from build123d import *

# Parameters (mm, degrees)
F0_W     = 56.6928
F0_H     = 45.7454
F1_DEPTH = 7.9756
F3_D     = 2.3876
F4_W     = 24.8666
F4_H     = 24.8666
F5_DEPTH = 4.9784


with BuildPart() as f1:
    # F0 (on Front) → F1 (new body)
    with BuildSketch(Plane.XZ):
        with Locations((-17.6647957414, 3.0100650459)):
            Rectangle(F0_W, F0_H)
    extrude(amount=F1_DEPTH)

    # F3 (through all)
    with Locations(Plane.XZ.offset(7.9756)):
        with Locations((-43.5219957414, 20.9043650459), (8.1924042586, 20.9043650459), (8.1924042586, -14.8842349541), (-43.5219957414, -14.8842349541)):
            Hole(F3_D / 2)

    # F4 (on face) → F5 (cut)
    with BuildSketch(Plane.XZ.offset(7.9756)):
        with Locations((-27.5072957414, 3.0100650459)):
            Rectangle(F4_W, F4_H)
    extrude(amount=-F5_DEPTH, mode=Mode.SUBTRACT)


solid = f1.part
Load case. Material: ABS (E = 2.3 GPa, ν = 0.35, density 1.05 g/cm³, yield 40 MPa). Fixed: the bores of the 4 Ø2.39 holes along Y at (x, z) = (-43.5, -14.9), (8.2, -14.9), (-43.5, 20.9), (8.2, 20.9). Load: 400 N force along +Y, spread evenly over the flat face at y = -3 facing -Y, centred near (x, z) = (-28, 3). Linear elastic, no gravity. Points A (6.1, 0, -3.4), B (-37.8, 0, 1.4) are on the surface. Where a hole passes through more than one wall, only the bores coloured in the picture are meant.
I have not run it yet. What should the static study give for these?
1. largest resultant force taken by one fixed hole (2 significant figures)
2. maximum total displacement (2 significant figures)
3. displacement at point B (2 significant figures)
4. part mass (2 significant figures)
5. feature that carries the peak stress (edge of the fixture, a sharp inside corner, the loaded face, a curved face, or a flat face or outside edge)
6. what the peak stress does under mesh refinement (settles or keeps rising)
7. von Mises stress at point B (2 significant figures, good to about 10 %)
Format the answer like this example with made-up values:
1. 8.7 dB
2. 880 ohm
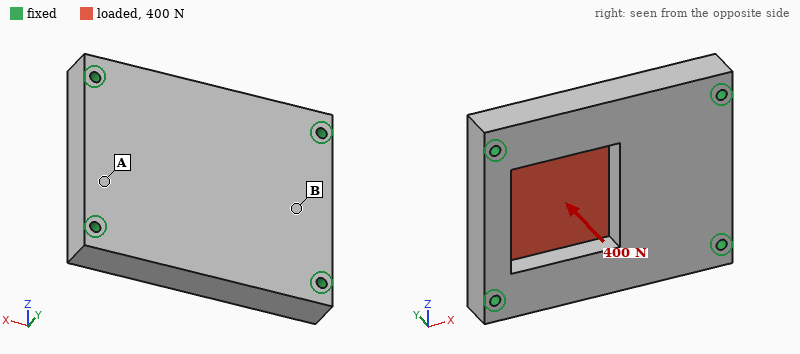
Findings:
1. 160 N
2. 0.25 mm
3. 0.12 mm
4. 18 g
5. edge of the fixture
6. keeps rising
7. 5.1 MPa
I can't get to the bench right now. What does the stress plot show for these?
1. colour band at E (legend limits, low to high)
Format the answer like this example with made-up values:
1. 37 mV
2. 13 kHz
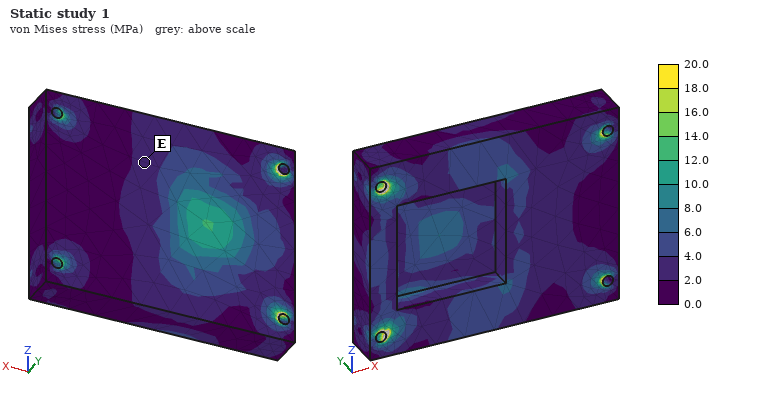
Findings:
1. 2.0 to 4.0 MPa
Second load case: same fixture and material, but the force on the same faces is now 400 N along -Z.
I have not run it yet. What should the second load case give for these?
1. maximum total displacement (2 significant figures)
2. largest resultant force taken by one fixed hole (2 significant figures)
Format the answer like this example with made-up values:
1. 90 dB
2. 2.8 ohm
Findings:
1. 33 µm
2. 130 N
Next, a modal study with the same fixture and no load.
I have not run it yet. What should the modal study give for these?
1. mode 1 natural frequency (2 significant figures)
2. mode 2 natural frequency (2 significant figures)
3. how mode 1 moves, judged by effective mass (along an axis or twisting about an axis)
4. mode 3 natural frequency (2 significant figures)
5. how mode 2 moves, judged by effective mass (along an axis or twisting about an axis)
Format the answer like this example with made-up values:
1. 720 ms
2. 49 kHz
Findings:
1. 2900 Hz
2. 4200 Hz
3. along Y
4. 6000 Hz
5. twisting about X
